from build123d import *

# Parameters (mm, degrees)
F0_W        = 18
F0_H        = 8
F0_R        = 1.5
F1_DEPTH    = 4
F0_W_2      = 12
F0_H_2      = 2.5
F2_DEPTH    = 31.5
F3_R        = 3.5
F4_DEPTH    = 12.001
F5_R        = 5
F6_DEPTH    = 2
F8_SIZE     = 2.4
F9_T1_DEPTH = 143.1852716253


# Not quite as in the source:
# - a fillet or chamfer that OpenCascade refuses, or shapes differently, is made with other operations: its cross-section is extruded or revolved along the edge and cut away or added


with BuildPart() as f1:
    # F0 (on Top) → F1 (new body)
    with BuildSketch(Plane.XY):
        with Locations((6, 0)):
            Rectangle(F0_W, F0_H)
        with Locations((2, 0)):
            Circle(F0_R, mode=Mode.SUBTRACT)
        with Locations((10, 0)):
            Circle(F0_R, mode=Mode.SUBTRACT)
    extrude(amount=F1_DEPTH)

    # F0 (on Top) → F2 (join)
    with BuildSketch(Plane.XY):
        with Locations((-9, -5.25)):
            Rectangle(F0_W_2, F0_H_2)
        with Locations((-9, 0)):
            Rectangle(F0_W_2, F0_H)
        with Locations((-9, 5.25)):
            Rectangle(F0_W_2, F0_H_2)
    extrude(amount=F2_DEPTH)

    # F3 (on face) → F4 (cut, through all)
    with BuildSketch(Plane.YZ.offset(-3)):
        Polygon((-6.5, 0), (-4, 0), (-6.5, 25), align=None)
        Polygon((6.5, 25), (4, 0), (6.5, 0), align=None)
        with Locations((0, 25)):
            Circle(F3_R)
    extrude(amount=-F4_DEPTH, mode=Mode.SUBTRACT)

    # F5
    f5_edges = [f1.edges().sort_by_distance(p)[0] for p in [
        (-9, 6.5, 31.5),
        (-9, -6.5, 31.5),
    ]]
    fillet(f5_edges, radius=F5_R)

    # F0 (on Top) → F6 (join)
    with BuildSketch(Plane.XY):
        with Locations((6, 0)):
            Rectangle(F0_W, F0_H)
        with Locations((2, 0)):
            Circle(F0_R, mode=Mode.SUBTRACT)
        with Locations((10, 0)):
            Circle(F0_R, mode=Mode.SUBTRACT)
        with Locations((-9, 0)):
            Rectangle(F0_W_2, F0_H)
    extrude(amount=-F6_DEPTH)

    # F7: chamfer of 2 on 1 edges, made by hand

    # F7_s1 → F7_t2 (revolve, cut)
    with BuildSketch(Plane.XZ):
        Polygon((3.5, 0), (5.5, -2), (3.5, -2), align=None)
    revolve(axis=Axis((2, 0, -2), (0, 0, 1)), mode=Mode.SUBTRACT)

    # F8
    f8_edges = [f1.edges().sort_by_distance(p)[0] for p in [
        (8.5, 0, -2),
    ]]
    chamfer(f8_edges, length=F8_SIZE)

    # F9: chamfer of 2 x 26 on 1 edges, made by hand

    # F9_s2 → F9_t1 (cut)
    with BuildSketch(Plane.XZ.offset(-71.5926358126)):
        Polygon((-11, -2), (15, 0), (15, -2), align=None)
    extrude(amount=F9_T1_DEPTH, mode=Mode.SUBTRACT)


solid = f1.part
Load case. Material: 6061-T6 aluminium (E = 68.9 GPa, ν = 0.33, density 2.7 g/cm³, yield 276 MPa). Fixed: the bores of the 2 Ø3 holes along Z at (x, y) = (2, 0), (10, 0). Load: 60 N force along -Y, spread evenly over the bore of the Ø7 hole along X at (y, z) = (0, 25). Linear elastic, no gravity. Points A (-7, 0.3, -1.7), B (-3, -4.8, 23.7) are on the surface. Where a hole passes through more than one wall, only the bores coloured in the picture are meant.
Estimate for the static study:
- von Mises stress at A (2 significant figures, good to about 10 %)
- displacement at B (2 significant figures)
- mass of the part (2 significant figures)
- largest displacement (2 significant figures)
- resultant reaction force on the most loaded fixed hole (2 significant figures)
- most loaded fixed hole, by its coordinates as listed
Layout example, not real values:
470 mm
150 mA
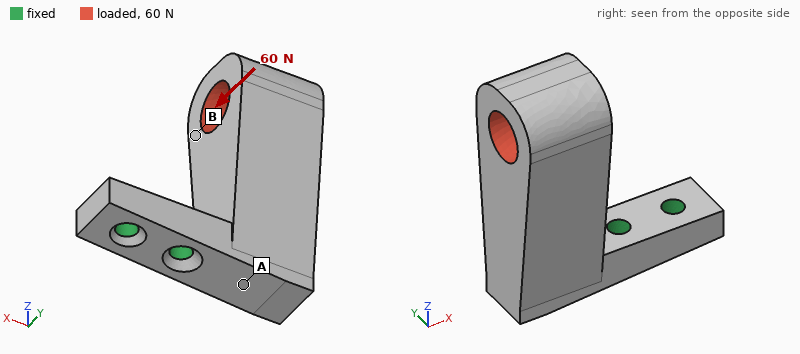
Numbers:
10 MPa
40 µm
12 g
57 µm
93 N
(2, 0)
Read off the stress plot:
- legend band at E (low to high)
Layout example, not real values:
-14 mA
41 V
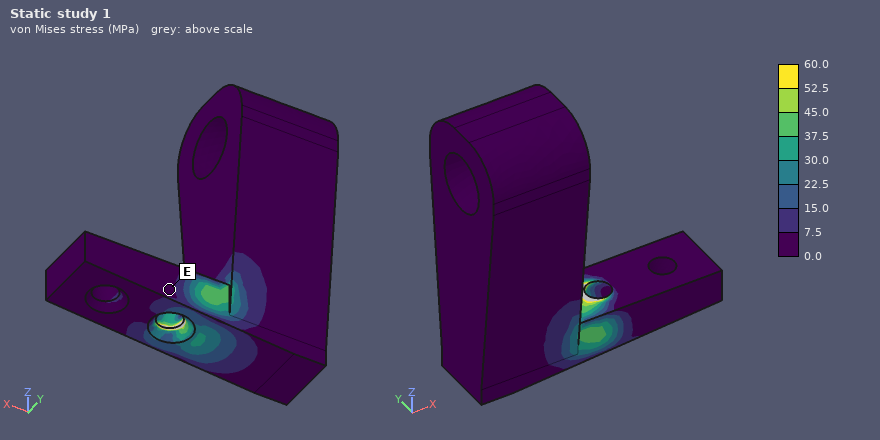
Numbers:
0.0 to 7.5 MPa
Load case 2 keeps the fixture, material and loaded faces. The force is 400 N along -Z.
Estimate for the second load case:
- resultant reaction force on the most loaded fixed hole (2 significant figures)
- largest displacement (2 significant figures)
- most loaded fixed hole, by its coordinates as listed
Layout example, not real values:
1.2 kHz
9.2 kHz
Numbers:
500 N
0.13 mm
(2, 0)
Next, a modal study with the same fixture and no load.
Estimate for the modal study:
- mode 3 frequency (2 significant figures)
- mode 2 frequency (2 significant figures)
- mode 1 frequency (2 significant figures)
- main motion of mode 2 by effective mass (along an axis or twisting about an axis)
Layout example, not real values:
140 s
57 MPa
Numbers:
8800 Hz
2600 Hz
2500 Hz
along Y
